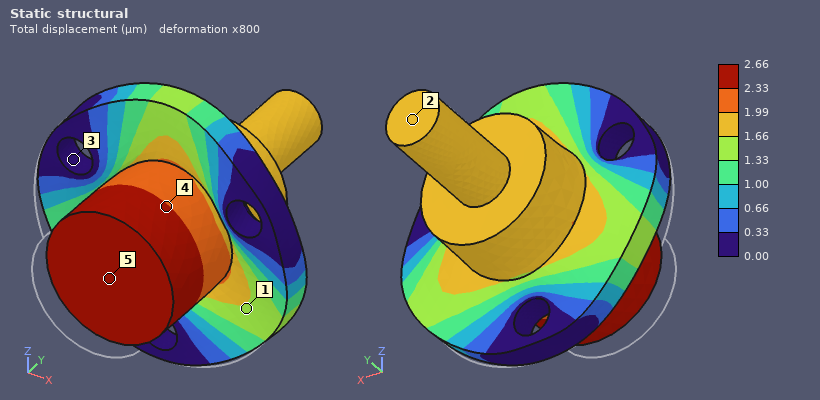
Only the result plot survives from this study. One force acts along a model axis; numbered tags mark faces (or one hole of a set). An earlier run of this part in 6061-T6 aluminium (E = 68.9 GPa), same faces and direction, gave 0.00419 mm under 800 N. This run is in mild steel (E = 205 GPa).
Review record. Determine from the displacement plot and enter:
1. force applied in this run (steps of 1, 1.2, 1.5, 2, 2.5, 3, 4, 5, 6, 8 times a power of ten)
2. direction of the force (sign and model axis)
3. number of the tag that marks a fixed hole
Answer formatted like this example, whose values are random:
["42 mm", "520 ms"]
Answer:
["1.5 kN", "+Y", "3"]
